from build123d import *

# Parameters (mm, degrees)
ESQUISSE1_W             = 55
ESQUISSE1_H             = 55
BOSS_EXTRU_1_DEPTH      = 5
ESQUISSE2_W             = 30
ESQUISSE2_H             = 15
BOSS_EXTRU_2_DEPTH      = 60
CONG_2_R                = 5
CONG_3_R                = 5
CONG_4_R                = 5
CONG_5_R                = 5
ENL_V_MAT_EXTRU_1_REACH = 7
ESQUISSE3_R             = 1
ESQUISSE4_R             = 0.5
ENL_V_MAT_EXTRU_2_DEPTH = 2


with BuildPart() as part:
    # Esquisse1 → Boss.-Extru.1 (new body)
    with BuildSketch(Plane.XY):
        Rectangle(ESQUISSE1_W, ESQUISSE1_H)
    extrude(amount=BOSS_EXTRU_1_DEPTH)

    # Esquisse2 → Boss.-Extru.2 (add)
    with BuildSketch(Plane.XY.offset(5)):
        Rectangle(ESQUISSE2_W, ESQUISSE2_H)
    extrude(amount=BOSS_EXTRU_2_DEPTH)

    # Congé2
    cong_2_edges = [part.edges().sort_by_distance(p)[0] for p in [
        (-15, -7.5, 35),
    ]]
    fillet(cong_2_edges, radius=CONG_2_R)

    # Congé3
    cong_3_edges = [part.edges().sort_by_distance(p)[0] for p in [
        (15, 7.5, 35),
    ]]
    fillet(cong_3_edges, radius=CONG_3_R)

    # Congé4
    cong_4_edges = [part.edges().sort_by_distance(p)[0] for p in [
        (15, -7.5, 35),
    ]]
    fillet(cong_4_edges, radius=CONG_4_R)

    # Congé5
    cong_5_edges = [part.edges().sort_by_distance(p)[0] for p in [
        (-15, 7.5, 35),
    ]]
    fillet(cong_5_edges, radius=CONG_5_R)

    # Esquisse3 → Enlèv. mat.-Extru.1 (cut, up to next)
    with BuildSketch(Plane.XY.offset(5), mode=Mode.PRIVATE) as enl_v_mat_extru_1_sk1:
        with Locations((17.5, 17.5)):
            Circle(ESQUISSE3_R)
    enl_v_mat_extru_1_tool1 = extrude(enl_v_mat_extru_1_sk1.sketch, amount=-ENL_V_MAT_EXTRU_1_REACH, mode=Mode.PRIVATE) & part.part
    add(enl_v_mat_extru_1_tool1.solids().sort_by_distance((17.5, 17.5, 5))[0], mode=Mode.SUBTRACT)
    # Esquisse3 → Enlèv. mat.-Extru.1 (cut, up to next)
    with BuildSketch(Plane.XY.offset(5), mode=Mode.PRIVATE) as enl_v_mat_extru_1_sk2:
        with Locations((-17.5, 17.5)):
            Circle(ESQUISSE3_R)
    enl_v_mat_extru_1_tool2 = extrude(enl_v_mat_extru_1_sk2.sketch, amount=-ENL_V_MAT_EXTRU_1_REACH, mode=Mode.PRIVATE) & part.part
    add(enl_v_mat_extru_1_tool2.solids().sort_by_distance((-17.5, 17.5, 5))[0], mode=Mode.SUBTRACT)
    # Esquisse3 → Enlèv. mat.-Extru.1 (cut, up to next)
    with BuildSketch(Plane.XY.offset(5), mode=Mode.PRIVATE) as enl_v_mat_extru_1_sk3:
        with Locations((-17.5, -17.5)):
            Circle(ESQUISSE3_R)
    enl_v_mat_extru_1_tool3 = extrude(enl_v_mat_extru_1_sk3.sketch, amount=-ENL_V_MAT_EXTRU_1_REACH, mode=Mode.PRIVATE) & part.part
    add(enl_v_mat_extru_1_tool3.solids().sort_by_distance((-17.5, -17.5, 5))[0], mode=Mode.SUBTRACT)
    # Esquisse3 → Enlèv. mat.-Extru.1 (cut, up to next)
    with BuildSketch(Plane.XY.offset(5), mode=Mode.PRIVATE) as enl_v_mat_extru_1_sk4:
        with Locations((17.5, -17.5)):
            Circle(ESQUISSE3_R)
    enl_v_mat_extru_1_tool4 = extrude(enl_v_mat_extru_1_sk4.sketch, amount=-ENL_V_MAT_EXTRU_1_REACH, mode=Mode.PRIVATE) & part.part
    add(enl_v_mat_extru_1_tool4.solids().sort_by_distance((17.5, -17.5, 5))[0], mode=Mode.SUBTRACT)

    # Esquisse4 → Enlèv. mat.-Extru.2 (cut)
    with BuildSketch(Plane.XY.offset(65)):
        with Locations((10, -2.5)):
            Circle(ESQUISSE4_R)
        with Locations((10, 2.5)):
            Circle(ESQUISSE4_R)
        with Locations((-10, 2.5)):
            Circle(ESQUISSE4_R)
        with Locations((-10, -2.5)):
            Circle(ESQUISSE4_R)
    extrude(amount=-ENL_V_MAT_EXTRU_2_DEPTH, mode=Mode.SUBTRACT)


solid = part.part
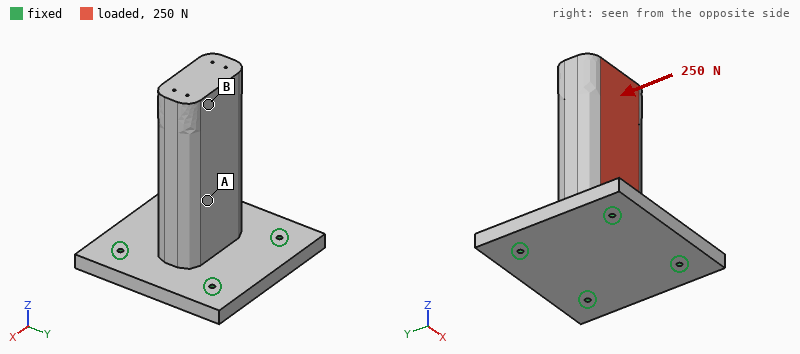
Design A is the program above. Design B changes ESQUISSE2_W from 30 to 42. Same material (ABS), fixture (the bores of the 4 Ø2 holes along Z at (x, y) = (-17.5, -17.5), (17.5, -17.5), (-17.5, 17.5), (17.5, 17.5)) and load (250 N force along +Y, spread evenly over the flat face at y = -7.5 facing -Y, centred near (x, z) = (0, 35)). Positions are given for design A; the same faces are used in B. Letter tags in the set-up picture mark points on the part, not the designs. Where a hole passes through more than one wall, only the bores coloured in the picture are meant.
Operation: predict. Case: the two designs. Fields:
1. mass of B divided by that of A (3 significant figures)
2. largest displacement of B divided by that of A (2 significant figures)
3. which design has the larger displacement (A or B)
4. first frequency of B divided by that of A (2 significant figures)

1.26
0.69
A
1.0
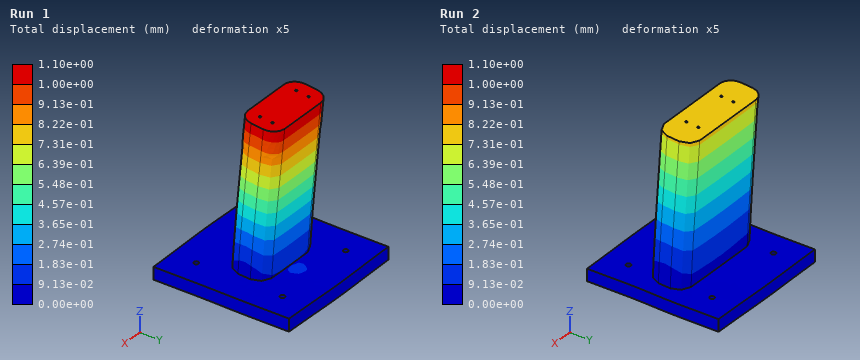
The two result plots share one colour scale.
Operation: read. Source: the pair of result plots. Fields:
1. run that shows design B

Run 2
